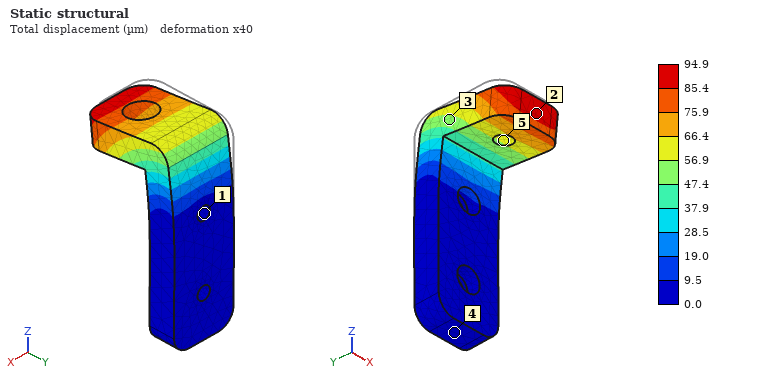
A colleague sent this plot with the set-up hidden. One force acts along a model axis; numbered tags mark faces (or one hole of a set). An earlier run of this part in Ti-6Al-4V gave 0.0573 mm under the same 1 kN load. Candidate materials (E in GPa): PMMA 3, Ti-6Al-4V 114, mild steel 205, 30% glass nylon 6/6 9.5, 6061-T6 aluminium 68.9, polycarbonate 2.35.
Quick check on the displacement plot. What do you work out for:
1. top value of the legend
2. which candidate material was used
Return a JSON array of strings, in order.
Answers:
["94.9 µm", "6061-T6 aluminium"]
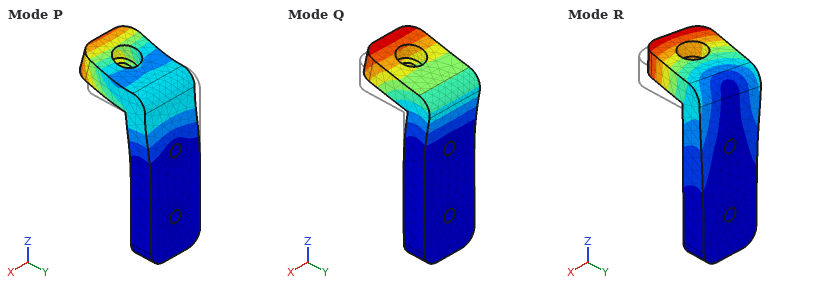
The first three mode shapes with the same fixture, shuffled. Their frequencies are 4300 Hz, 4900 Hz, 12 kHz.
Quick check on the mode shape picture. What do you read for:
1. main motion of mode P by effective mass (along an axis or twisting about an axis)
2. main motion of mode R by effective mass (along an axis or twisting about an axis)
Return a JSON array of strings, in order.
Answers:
["along Y", "along X"]
